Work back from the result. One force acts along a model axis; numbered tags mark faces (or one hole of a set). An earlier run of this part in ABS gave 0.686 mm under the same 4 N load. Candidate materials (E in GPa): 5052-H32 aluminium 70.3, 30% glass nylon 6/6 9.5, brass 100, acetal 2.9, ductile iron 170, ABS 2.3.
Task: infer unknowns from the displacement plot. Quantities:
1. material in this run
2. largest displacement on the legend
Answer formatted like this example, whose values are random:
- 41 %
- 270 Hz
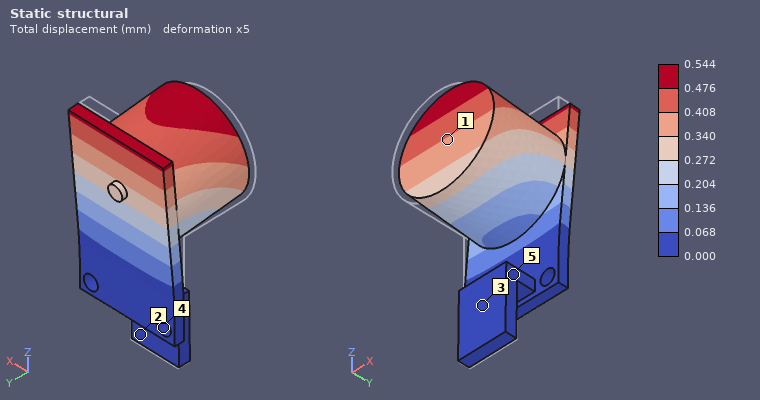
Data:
- acetal
- 0.544 mm
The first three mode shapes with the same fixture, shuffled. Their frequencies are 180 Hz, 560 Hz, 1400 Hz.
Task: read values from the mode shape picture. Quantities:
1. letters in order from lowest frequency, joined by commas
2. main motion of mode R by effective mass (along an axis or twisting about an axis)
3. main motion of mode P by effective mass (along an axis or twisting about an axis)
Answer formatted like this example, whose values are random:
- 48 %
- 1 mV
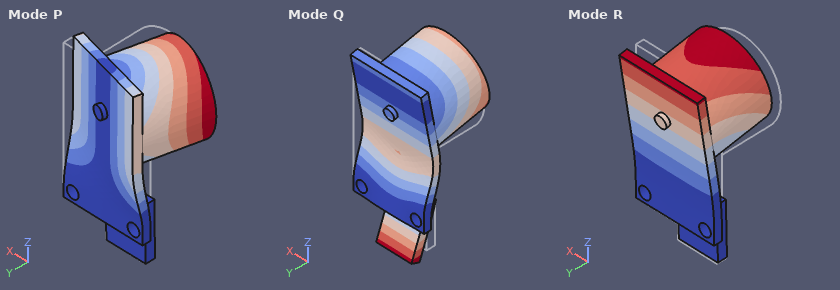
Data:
- R, P, Q
- along Y
- along X
